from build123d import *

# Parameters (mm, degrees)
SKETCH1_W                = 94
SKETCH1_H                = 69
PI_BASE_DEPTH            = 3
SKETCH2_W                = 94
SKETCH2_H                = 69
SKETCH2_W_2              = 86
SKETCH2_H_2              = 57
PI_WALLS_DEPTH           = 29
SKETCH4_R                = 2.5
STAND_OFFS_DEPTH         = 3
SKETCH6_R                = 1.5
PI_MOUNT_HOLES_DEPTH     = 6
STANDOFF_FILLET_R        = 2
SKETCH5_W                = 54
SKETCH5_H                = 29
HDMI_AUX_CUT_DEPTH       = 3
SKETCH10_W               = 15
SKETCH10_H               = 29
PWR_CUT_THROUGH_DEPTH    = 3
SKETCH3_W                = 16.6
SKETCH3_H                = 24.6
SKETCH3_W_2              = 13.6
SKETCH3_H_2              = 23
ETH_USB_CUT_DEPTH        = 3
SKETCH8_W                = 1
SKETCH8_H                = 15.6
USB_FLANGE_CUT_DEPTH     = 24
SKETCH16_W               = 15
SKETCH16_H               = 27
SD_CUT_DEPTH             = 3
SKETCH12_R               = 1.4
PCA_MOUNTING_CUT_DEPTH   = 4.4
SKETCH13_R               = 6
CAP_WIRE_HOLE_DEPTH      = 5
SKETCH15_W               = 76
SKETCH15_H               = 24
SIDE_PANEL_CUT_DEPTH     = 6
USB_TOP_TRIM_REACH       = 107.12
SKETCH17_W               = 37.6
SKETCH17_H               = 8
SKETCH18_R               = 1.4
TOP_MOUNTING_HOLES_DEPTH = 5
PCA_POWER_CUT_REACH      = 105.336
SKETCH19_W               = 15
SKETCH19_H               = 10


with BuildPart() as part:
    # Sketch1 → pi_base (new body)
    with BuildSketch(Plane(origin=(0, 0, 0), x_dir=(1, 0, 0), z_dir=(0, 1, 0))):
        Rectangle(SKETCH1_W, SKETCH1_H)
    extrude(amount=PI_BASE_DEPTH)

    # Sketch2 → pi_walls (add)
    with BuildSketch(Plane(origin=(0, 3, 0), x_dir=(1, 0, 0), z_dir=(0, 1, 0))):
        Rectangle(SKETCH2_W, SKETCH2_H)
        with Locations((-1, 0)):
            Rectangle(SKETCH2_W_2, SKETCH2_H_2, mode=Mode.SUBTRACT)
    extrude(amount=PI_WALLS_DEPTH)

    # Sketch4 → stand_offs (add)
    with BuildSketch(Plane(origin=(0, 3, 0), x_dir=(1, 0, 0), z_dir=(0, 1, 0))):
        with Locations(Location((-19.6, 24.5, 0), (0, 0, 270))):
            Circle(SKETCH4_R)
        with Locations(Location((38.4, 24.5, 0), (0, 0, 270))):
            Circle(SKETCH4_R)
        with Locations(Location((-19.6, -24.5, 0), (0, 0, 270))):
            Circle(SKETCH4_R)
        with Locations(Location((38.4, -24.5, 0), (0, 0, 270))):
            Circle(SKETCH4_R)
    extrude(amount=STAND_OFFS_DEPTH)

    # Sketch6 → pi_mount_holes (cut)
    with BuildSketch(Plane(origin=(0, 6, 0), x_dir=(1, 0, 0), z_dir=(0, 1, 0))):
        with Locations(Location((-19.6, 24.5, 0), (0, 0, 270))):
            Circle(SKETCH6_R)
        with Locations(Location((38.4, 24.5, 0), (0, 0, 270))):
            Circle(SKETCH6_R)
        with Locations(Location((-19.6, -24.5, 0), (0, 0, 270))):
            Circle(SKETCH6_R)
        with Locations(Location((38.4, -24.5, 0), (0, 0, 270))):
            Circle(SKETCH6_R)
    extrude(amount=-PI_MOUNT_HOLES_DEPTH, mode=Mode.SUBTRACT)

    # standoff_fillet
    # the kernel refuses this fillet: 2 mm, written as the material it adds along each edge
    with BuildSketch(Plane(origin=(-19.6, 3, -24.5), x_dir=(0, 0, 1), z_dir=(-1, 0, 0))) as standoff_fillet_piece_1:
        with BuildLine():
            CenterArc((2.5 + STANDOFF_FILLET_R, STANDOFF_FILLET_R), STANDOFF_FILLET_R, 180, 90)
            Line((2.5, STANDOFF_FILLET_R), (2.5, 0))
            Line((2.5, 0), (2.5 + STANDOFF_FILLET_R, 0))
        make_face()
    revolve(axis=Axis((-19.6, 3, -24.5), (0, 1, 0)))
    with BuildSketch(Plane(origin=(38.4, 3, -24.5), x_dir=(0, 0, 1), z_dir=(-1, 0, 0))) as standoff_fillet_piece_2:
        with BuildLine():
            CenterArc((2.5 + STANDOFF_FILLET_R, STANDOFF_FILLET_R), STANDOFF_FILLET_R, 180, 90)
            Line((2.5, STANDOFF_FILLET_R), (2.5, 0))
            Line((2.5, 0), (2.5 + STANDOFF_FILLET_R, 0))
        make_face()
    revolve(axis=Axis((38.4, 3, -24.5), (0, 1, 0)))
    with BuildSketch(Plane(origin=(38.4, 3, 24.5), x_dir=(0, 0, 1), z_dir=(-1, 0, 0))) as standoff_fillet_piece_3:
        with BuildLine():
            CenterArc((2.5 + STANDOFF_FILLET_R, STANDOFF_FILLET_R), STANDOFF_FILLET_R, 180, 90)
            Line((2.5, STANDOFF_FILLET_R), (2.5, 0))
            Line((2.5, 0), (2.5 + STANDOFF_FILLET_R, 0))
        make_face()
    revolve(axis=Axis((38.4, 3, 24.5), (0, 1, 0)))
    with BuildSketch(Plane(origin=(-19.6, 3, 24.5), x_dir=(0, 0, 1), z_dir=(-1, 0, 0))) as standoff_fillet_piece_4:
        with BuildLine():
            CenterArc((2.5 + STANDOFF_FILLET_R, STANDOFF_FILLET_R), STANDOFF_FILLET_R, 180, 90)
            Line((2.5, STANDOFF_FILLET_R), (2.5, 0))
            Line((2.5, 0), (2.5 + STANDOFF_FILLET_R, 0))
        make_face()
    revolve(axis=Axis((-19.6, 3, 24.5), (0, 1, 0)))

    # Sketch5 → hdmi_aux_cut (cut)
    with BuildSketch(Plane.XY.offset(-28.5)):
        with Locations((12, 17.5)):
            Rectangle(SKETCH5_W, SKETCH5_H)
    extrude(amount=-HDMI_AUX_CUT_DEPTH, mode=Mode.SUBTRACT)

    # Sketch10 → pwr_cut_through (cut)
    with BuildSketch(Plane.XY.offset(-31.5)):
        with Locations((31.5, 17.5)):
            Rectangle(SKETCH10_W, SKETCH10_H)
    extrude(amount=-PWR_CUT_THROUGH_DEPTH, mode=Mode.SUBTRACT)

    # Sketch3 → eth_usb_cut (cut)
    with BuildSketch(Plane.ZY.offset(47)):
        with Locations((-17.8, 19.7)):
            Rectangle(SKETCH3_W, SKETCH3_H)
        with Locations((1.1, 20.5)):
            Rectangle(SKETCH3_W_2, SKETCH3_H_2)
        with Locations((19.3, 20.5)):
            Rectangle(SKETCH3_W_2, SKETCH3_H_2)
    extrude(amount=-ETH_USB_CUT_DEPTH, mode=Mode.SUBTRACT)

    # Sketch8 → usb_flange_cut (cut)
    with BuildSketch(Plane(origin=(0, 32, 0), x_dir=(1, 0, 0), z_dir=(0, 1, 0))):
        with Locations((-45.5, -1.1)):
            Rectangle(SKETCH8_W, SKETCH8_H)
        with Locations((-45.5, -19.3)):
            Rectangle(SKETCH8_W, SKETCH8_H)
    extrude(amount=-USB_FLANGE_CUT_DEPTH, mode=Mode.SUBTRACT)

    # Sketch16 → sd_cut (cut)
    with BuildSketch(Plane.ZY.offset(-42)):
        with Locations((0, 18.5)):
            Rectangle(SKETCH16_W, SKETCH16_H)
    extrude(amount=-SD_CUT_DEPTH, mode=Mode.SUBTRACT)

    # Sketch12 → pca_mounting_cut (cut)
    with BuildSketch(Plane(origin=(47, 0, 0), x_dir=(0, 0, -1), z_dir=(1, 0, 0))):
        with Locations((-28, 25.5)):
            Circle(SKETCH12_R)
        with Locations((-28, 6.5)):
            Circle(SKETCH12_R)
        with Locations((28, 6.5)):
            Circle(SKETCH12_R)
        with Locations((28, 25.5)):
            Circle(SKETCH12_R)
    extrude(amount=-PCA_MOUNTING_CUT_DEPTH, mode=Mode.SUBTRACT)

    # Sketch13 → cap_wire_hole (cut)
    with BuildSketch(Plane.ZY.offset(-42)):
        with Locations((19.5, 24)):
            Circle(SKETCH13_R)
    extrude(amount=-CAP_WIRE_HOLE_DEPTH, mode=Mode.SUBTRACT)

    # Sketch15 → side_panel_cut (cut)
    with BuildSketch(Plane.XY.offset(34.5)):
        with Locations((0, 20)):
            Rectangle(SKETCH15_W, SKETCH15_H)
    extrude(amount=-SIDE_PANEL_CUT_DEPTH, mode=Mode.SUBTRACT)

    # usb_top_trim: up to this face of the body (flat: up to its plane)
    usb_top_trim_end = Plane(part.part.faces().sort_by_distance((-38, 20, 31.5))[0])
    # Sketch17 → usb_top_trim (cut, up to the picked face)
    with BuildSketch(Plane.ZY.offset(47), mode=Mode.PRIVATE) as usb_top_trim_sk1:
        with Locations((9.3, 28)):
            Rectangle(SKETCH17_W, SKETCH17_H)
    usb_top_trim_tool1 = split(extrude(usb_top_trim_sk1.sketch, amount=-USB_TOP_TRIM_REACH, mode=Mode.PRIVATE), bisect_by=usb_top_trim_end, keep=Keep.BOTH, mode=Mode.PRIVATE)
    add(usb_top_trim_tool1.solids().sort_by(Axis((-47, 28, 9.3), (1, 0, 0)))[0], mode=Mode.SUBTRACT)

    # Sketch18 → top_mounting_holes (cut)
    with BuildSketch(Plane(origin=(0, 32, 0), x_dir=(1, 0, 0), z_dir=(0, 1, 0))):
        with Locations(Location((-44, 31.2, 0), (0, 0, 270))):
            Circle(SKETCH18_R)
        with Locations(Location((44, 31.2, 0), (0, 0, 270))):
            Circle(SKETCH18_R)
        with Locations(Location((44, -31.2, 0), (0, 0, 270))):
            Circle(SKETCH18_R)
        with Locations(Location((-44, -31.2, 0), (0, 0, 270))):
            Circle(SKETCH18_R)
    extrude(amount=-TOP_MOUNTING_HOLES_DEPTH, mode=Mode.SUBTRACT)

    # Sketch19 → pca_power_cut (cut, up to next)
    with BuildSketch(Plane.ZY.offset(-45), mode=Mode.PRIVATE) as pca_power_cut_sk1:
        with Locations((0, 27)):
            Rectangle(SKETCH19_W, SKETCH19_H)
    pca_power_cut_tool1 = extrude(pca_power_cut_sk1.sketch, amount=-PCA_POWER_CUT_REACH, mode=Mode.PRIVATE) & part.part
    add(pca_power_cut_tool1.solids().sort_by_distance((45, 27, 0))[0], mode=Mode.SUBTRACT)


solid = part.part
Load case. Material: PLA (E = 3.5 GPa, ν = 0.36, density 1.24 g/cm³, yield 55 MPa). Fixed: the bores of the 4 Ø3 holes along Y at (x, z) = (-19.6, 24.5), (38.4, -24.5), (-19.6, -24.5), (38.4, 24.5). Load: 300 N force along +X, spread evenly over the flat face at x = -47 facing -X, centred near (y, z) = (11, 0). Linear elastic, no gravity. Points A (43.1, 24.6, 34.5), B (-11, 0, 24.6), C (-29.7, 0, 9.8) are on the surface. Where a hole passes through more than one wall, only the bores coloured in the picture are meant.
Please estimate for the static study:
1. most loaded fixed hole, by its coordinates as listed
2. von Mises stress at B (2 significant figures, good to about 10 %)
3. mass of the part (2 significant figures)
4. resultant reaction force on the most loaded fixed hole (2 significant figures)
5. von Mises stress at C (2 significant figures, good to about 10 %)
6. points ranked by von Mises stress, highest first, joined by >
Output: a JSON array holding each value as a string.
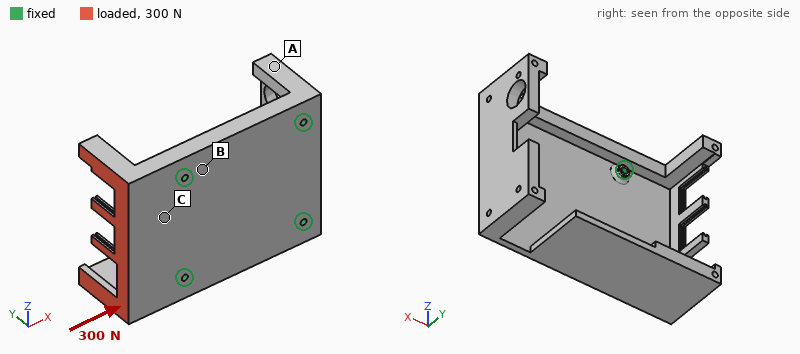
["(-19.6, -24.5)", "3.3 MPa", "53 g", "120 N", "4.6 MPa", "C > B > A"]
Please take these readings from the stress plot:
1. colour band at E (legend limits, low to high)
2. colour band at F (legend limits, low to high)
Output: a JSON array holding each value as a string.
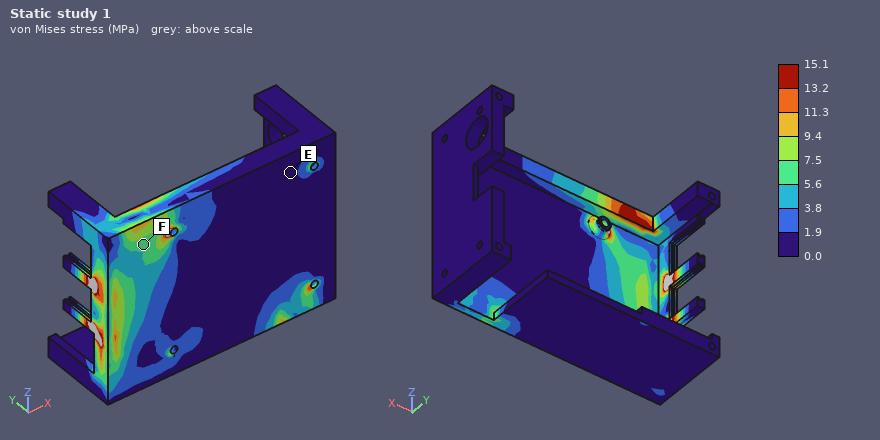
["0.0 to 1.9 MPa", "5.6 to 7.5 MPa"]
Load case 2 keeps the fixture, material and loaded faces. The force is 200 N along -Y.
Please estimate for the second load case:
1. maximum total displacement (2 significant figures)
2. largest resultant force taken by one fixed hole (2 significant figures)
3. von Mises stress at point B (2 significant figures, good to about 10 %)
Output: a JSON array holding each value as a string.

["1.3 mm", "160 N", "3.8 MPa"]
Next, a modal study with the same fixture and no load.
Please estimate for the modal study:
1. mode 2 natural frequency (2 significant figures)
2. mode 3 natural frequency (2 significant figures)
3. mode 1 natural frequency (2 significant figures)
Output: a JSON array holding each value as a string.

["870 Hz", "910 Hz", "680 Hz"]
